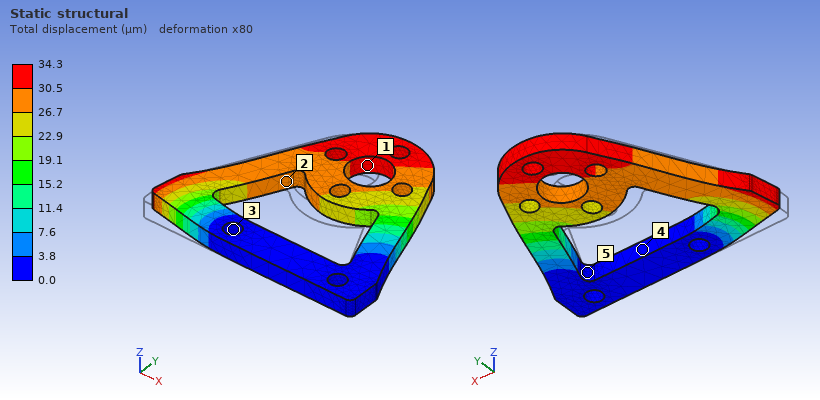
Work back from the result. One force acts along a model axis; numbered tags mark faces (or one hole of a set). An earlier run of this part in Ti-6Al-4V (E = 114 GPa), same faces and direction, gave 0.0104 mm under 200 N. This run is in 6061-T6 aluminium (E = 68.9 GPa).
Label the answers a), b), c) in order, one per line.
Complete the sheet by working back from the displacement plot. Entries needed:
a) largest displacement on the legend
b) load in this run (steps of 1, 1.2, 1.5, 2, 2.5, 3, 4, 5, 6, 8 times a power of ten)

a) 34.3 µm
b) 400 N
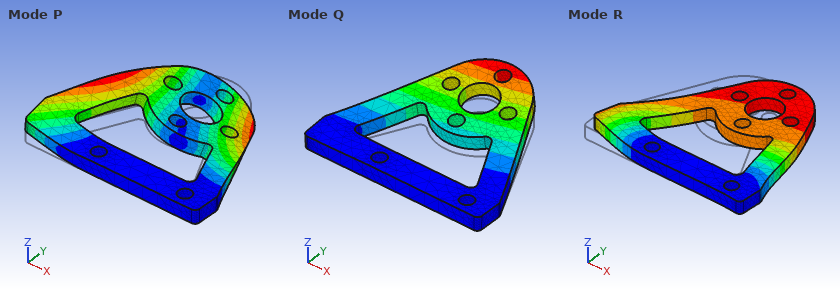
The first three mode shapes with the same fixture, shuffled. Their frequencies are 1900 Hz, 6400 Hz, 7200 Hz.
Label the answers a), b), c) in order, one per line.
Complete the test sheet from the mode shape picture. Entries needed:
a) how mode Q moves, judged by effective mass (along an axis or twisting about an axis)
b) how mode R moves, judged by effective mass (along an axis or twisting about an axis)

a) along Z
b) along X
